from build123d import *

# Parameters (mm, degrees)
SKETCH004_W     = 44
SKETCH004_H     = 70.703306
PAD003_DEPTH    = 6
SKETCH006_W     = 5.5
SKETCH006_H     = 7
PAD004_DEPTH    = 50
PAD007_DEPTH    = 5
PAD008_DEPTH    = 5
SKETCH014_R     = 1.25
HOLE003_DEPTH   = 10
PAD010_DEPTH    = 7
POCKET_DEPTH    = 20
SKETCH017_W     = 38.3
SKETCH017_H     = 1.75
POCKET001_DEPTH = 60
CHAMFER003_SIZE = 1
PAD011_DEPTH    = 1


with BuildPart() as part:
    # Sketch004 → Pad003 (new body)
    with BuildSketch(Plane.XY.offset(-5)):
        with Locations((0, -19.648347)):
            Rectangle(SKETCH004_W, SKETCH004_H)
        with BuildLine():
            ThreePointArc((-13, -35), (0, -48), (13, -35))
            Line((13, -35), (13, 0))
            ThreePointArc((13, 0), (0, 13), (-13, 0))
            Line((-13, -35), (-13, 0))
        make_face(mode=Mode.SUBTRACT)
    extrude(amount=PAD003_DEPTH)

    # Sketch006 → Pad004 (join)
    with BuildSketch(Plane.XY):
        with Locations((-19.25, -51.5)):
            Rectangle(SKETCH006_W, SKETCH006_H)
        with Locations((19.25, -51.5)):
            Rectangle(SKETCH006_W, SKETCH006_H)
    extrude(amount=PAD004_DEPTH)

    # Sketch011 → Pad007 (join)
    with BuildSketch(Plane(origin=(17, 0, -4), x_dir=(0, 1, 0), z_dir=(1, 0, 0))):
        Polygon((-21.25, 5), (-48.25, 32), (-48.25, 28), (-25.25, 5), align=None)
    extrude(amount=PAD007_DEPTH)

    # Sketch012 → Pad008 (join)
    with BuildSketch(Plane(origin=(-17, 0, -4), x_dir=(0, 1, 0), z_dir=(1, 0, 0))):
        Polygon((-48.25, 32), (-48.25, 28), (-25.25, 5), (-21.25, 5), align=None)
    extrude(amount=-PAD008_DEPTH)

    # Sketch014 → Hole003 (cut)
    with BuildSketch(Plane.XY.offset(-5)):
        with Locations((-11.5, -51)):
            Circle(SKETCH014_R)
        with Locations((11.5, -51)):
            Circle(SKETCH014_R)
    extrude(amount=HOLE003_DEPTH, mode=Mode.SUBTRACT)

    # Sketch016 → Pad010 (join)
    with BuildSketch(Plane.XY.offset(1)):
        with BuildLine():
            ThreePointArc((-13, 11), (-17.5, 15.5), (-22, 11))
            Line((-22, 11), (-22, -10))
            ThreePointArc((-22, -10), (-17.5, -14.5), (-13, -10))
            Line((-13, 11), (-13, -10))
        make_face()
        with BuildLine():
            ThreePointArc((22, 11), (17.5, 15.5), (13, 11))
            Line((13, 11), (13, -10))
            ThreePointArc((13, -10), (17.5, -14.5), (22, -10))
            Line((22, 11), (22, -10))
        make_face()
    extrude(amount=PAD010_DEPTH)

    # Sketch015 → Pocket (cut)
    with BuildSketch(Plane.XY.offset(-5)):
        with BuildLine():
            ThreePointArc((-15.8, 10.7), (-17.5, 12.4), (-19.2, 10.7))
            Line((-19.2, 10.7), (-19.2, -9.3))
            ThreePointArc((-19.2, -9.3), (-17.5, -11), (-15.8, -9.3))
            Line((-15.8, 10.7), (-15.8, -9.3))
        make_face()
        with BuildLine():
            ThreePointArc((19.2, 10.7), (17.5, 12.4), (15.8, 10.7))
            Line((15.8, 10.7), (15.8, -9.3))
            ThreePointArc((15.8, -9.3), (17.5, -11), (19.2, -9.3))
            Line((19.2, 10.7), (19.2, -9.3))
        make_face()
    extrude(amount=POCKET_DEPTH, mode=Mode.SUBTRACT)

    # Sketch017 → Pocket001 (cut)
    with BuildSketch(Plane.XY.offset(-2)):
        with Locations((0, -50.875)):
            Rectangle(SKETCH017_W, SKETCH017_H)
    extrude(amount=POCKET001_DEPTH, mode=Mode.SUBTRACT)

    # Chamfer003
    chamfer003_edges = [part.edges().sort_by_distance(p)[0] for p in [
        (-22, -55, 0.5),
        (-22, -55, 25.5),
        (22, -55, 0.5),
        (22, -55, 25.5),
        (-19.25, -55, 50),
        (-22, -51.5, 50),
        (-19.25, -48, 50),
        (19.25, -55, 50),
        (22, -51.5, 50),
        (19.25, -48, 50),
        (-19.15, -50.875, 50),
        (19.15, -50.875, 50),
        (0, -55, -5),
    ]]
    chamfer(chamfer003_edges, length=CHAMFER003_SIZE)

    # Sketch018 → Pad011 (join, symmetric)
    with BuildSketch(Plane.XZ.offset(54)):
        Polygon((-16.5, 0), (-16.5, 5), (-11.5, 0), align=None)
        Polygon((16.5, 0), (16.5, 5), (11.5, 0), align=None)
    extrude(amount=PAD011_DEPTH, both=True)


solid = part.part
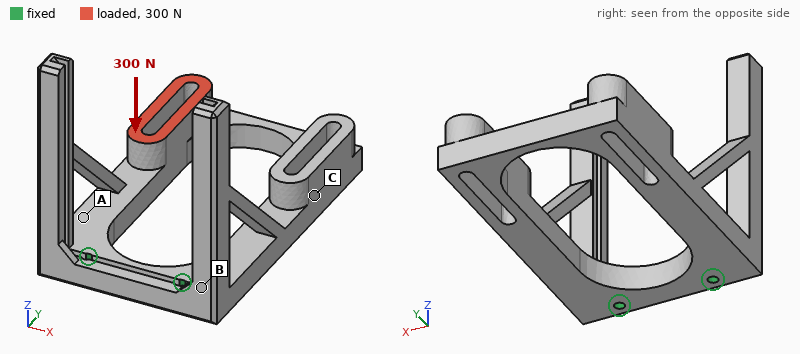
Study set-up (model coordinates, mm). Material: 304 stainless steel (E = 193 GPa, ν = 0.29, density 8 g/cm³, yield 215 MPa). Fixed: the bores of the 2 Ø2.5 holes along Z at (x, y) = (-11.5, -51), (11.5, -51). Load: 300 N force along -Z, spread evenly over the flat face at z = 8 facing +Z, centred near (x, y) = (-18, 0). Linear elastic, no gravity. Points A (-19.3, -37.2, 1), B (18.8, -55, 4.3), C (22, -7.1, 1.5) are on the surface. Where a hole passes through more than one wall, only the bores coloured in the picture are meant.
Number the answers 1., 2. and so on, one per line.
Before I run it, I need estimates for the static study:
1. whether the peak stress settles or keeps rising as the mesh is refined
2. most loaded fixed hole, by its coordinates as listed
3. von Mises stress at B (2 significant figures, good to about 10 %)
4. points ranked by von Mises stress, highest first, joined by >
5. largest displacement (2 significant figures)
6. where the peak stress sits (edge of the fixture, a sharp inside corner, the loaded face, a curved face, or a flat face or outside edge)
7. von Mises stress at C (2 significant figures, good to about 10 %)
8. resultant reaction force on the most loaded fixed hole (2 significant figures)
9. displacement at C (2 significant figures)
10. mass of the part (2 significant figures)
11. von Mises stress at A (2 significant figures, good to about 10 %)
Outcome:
1. keeps rising
2. (-11.5, -51)
3. 40 MPa
4. A > B > C
5. 0.30 mm
6. edge of the fixture
7. 20 MPa
8. 280 N
9. 0.088 mm
10. 120 g
11. 74 MPa
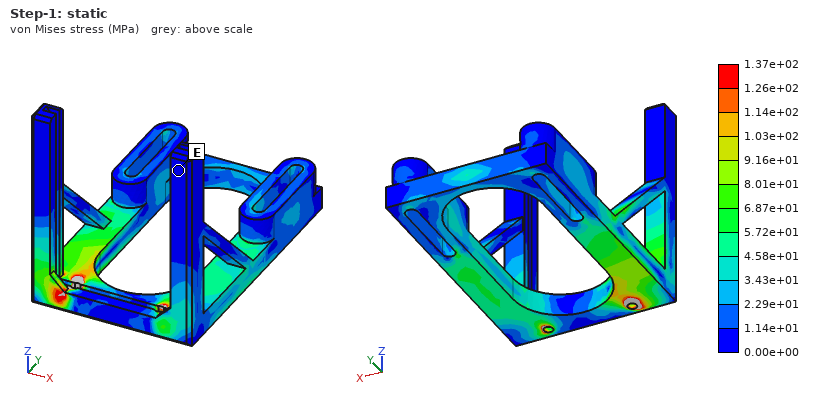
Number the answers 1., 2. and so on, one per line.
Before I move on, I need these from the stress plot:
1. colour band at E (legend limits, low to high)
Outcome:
1. 0.00e+00 to 1.14e+01 MPa
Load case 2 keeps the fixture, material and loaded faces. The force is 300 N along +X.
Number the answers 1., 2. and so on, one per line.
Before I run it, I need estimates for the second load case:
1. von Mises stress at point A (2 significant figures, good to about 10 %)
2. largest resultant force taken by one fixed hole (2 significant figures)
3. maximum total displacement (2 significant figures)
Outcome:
1. 35 MPa
2. 510 N
3. 0.10 mm
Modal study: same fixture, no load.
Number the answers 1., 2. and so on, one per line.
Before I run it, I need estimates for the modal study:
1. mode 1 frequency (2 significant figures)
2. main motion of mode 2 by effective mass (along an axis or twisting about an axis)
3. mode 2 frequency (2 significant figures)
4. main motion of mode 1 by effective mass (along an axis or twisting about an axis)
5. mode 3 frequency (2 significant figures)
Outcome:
1. 860 Hz
2. along X
3. 1500 Hz
4. along Z
5. 1600 Hz
